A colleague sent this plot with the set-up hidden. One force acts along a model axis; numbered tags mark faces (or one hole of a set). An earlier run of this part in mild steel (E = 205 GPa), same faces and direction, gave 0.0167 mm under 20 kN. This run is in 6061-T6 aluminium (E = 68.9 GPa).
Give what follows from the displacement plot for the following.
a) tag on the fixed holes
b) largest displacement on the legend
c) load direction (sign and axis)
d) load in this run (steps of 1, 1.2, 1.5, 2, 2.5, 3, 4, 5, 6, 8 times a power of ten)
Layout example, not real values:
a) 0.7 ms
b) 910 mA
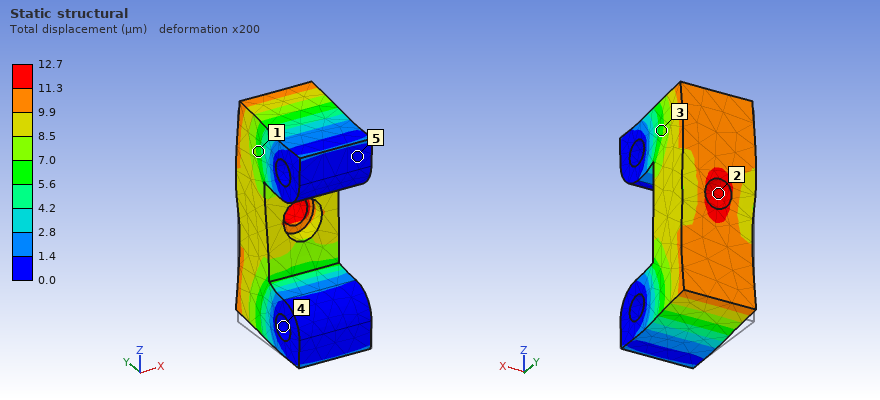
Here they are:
a) 4
b) 12.7 µm
c) +Z
d) 5 kN
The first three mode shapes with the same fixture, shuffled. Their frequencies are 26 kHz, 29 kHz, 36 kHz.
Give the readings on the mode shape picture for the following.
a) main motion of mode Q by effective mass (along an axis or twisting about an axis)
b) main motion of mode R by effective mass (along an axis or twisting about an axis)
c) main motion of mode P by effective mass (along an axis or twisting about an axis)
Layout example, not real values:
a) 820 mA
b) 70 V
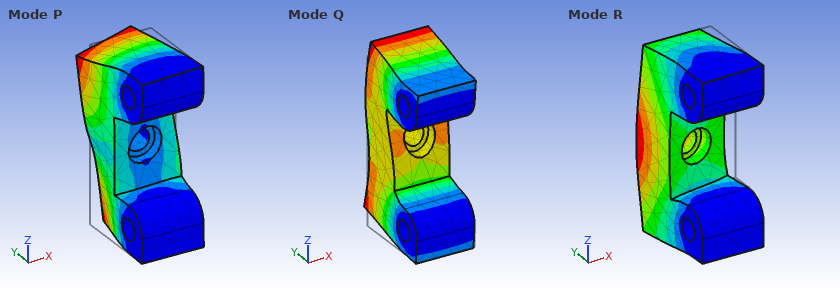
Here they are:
a) along Z
b) along X
c) twisting about Y
